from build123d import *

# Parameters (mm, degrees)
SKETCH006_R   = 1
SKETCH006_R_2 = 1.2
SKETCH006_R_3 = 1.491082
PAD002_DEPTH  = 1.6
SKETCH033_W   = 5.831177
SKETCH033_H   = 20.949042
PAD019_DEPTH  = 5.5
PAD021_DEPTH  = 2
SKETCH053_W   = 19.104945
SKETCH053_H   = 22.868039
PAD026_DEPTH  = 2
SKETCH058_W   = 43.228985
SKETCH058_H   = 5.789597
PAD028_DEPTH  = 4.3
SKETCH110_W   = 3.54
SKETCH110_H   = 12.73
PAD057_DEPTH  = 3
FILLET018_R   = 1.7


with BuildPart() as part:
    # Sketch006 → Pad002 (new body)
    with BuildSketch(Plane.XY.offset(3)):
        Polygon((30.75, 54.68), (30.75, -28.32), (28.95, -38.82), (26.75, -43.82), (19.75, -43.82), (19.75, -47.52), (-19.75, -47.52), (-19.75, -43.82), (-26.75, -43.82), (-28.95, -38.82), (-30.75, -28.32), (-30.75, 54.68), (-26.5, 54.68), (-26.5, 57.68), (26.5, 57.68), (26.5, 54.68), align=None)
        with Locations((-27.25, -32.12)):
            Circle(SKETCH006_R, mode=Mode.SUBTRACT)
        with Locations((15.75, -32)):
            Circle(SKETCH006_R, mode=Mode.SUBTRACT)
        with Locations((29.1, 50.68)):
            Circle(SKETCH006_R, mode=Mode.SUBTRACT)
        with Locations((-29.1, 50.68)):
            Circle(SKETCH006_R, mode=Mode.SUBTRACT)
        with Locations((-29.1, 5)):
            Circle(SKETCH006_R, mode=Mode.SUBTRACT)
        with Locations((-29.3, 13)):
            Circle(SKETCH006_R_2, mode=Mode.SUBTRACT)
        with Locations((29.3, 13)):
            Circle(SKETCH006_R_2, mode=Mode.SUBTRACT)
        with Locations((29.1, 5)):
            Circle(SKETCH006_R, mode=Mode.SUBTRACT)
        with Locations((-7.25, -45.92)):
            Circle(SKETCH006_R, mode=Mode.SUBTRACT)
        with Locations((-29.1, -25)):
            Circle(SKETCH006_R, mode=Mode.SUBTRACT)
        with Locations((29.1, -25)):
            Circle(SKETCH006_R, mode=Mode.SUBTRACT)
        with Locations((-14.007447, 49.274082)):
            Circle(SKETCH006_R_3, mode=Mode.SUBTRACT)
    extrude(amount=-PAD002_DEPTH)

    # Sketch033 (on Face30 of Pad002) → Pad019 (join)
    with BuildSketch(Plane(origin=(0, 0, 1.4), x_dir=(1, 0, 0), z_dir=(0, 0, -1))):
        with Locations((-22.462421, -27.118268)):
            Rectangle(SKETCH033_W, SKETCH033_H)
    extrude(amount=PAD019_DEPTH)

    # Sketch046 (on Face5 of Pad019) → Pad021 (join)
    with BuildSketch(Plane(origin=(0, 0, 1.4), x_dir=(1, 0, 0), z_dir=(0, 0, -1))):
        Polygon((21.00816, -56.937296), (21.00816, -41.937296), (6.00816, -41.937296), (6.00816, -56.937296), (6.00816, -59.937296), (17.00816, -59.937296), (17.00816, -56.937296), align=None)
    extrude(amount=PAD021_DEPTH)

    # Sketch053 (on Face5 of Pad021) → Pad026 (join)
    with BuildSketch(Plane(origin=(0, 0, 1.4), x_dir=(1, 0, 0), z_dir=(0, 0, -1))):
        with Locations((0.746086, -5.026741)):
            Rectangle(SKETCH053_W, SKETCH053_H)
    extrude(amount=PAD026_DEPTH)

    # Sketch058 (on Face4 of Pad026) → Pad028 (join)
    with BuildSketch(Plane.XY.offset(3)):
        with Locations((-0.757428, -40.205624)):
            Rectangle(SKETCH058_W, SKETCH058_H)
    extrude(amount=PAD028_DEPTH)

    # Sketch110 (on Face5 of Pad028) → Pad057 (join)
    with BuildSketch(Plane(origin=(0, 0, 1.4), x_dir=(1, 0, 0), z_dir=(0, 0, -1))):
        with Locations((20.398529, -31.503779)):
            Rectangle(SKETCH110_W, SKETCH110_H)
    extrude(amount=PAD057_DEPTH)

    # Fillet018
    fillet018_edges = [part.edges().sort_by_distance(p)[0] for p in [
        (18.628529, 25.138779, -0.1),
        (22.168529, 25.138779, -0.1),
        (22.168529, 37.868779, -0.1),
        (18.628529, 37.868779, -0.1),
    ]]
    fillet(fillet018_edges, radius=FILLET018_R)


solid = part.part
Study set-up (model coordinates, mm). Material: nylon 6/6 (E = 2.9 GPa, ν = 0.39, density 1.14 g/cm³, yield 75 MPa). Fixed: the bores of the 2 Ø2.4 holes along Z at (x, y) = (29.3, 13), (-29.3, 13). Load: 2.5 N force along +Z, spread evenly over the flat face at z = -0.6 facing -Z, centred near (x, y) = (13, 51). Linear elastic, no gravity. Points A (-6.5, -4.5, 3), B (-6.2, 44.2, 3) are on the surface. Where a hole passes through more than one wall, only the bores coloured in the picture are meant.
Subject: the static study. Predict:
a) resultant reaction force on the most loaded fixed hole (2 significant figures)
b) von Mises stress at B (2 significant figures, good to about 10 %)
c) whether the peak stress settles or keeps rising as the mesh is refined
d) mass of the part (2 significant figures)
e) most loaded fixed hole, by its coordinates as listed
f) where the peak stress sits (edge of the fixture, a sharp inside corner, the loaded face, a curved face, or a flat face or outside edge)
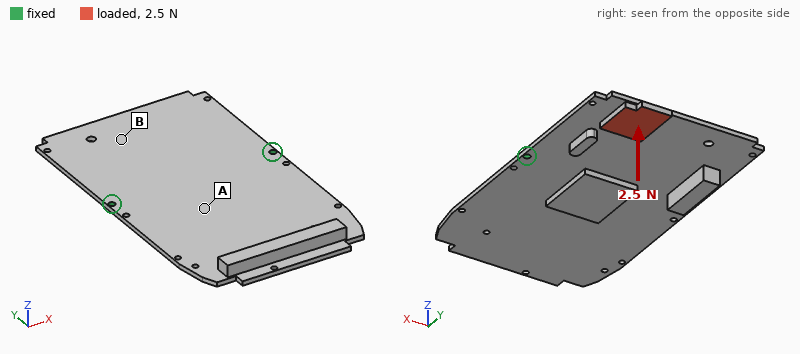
2.0 N
1.4 MPa
keeps rising
15 g
(29.3, 13)
edge of the fixture
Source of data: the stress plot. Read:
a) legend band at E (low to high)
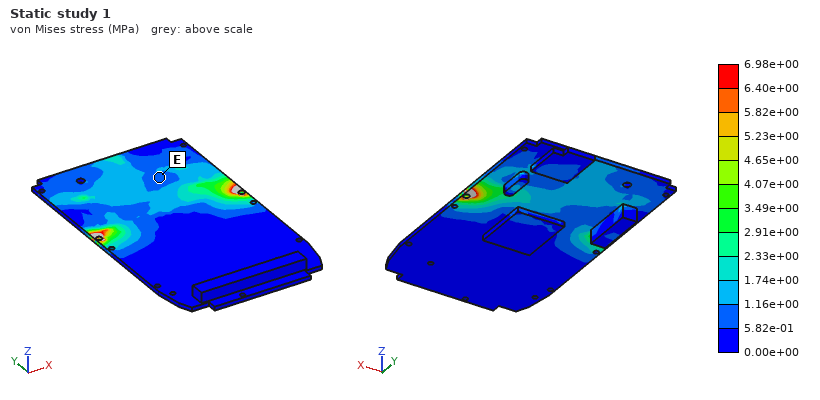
5.82e-01 to 1.16e+00 MPa
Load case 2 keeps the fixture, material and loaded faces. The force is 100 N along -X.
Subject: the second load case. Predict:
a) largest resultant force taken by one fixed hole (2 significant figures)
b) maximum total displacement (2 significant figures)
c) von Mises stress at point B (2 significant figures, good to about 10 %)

84 N
1.4 mm
4.0 MPa
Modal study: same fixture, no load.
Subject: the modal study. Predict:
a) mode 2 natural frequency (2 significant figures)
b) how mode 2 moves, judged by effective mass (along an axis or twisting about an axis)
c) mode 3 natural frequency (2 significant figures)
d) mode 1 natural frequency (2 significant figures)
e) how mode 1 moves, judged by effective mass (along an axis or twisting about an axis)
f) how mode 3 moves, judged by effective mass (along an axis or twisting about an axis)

190 Hz
along Z
330 Hz
81 Hz
along Z
twisting about Y
